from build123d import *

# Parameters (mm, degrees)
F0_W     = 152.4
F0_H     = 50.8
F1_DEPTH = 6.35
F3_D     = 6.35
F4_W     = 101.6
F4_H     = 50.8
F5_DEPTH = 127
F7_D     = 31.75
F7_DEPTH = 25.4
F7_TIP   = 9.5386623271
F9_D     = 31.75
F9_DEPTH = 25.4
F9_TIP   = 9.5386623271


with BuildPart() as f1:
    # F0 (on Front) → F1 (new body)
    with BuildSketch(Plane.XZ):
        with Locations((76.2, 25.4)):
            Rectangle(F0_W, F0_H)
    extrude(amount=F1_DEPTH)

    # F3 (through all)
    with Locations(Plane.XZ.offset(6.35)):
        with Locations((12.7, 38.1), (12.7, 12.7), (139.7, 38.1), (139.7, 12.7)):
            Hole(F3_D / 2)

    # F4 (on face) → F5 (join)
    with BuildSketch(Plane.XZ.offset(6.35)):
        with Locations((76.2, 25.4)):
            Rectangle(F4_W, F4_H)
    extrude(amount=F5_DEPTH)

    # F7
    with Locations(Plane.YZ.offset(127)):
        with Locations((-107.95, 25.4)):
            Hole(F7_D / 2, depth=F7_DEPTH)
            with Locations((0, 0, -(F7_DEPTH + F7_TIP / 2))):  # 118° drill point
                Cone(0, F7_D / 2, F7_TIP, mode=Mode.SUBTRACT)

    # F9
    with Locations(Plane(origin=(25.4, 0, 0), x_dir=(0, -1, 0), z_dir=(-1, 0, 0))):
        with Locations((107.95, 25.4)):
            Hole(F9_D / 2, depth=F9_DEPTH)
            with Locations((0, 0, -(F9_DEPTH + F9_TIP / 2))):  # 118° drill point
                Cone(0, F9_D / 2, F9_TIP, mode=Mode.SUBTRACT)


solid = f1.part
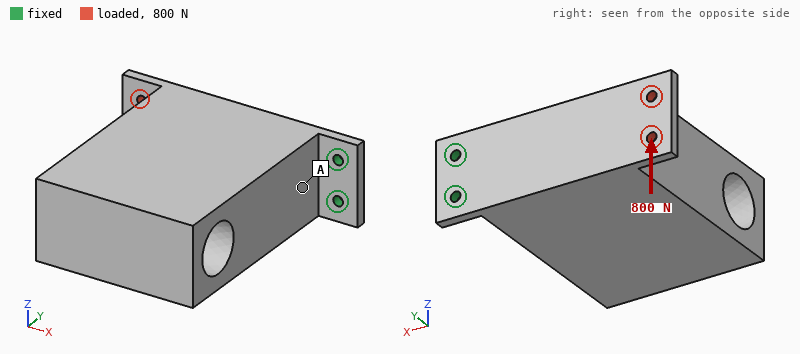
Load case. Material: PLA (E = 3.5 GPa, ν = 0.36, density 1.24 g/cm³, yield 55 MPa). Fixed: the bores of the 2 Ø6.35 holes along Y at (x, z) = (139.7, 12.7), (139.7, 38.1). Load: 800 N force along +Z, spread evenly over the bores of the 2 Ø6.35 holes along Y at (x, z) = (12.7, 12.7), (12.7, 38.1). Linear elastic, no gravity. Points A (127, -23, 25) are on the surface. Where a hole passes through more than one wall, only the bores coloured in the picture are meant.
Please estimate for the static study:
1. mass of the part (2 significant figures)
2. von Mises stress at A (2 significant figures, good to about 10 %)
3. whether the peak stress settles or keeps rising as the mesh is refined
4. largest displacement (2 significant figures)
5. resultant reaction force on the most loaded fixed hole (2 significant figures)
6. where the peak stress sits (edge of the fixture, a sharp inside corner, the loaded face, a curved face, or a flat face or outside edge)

820 g
5.0 MPa
keeps rising
2.1 mm
3.5 kN
edge of the fixture
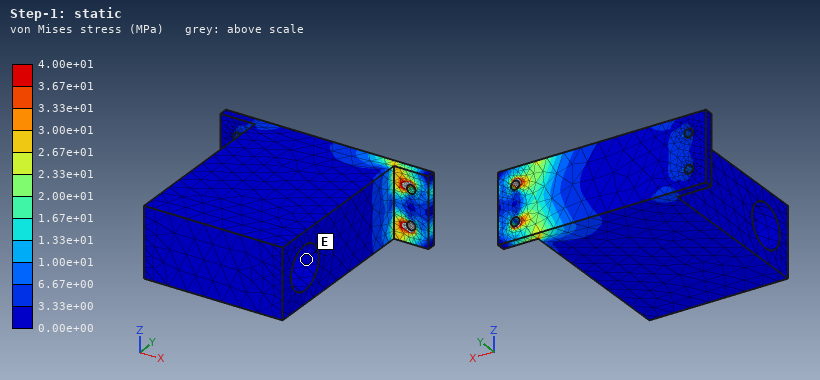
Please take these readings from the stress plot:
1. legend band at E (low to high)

0.00e+00 to 3.33e+00 MPa
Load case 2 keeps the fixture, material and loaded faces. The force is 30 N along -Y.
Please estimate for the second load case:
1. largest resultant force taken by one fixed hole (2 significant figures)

15 N
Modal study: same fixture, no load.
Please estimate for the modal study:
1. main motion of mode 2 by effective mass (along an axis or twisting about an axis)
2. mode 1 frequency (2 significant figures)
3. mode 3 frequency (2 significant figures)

along Z
30 Hz
310 Hz
